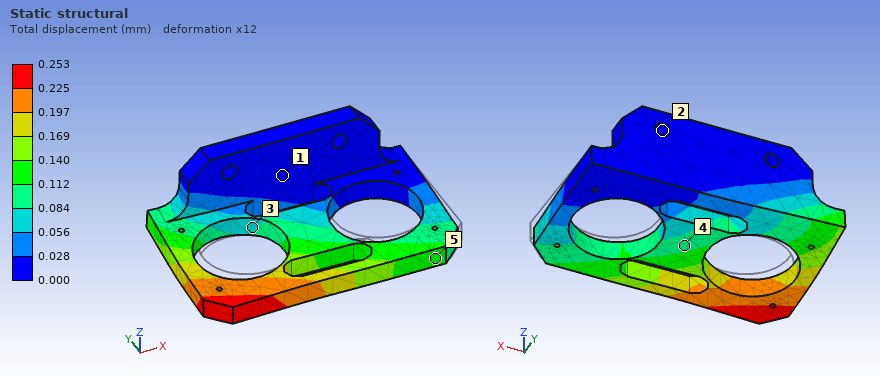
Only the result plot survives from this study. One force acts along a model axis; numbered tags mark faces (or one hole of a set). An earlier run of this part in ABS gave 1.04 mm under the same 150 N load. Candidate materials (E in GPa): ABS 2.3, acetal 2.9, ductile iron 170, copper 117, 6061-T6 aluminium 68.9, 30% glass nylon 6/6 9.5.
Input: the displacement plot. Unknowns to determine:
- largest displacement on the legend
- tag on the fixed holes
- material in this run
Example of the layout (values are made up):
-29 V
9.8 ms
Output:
0.253 mm
2
30% glass nylon 6/6
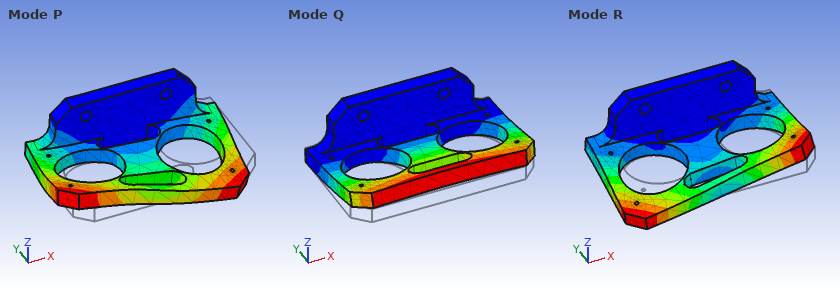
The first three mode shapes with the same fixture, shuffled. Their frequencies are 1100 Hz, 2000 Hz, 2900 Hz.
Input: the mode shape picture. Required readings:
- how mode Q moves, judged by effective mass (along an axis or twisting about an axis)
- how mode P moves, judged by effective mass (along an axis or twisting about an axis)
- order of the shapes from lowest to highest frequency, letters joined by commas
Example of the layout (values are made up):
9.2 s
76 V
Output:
along Z
along X
Q, R, P
